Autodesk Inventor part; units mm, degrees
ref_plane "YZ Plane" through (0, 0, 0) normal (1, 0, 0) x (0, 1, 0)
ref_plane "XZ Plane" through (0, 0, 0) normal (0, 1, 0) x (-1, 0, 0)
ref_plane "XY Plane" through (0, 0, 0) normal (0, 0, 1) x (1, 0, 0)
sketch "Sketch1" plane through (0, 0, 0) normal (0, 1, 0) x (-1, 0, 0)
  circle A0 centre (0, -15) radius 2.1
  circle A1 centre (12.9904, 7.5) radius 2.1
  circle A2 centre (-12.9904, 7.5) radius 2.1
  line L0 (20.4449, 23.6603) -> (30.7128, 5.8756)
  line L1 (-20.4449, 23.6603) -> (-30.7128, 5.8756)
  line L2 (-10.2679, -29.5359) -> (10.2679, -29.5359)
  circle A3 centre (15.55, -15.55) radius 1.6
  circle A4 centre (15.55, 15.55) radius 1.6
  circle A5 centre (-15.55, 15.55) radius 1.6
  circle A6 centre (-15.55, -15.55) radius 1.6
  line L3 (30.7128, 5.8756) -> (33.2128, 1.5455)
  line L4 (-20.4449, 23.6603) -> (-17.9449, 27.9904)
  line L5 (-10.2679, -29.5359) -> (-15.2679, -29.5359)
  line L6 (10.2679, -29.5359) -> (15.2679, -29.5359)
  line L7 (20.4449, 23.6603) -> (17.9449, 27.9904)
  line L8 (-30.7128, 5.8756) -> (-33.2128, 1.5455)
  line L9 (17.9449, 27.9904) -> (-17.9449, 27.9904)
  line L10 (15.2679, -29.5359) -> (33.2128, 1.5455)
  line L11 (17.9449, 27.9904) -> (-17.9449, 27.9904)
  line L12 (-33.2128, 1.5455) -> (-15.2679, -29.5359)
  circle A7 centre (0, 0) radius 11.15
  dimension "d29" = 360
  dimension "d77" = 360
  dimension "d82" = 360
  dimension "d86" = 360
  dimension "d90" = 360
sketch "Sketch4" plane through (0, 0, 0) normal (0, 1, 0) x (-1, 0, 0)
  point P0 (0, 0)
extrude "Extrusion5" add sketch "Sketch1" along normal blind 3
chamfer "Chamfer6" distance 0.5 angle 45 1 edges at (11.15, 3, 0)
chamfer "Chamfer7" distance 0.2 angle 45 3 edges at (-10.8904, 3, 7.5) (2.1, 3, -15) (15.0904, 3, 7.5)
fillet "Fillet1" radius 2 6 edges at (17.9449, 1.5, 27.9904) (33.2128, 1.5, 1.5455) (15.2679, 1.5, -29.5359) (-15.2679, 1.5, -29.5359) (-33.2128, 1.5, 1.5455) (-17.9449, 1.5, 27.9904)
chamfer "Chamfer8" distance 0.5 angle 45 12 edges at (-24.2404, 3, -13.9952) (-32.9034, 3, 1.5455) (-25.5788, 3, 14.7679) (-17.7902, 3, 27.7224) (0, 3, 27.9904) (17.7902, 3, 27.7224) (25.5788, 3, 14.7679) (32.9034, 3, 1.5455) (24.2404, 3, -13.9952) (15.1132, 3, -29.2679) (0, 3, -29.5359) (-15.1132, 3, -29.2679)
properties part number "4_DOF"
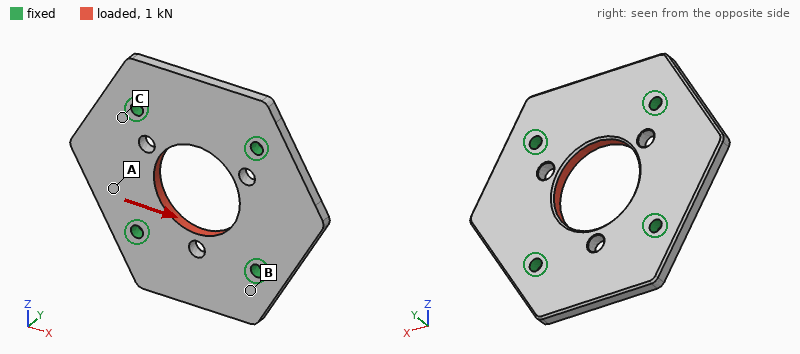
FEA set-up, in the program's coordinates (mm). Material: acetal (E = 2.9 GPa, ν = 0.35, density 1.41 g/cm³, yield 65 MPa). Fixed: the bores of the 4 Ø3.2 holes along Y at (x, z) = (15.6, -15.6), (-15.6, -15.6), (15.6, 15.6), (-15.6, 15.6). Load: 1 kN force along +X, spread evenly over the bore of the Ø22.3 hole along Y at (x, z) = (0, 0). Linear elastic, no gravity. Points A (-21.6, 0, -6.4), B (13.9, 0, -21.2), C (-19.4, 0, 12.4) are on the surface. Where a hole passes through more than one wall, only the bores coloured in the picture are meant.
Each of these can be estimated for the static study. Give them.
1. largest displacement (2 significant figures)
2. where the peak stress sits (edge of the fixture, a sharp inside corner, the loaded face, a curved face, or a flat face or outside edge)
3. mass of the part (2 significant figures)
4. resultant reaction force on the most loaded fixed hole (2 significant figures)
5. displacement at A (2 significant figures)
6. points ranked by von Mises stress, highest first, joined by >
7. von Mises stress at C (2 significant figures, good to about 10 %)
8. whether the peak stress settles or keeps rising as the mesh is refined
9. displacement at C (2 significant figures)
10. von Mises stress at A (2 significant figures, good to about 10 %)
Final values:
58 µm
edge of the fixture
10 g
250 N
34 µm
C > A > B
5.9 MPa
keeps rising
13 µm
3.2 MPa
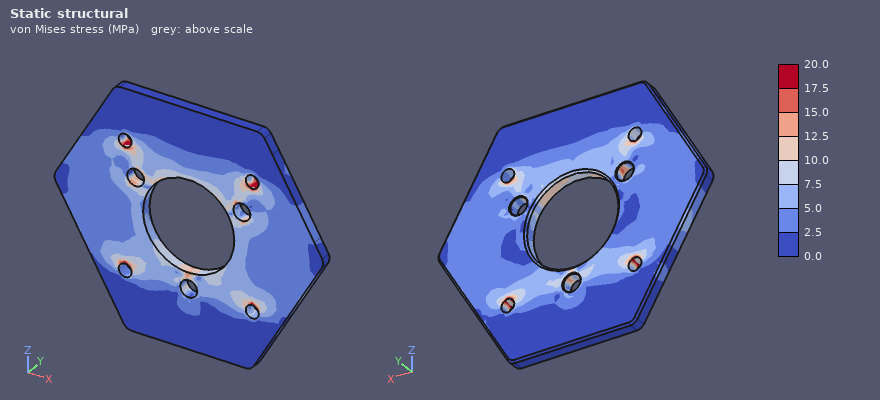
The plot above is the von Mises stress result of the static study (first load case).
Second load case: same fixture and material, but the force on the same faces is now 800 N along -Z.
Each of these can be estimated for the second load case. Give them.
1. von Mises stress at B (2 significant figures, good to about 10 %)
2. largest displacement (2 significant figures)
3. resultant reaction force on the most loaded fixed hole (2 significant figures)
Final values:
3.6 MPa
54 µm
210 N
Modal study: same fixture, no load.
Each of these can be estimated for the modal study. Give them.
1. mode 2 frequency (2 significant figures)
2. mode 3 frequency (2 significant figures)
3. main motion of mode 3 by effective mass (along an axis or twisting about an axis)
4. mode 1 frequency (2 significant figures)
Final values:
2500 Hz
2800 Hz
along Y
2500 Hz
